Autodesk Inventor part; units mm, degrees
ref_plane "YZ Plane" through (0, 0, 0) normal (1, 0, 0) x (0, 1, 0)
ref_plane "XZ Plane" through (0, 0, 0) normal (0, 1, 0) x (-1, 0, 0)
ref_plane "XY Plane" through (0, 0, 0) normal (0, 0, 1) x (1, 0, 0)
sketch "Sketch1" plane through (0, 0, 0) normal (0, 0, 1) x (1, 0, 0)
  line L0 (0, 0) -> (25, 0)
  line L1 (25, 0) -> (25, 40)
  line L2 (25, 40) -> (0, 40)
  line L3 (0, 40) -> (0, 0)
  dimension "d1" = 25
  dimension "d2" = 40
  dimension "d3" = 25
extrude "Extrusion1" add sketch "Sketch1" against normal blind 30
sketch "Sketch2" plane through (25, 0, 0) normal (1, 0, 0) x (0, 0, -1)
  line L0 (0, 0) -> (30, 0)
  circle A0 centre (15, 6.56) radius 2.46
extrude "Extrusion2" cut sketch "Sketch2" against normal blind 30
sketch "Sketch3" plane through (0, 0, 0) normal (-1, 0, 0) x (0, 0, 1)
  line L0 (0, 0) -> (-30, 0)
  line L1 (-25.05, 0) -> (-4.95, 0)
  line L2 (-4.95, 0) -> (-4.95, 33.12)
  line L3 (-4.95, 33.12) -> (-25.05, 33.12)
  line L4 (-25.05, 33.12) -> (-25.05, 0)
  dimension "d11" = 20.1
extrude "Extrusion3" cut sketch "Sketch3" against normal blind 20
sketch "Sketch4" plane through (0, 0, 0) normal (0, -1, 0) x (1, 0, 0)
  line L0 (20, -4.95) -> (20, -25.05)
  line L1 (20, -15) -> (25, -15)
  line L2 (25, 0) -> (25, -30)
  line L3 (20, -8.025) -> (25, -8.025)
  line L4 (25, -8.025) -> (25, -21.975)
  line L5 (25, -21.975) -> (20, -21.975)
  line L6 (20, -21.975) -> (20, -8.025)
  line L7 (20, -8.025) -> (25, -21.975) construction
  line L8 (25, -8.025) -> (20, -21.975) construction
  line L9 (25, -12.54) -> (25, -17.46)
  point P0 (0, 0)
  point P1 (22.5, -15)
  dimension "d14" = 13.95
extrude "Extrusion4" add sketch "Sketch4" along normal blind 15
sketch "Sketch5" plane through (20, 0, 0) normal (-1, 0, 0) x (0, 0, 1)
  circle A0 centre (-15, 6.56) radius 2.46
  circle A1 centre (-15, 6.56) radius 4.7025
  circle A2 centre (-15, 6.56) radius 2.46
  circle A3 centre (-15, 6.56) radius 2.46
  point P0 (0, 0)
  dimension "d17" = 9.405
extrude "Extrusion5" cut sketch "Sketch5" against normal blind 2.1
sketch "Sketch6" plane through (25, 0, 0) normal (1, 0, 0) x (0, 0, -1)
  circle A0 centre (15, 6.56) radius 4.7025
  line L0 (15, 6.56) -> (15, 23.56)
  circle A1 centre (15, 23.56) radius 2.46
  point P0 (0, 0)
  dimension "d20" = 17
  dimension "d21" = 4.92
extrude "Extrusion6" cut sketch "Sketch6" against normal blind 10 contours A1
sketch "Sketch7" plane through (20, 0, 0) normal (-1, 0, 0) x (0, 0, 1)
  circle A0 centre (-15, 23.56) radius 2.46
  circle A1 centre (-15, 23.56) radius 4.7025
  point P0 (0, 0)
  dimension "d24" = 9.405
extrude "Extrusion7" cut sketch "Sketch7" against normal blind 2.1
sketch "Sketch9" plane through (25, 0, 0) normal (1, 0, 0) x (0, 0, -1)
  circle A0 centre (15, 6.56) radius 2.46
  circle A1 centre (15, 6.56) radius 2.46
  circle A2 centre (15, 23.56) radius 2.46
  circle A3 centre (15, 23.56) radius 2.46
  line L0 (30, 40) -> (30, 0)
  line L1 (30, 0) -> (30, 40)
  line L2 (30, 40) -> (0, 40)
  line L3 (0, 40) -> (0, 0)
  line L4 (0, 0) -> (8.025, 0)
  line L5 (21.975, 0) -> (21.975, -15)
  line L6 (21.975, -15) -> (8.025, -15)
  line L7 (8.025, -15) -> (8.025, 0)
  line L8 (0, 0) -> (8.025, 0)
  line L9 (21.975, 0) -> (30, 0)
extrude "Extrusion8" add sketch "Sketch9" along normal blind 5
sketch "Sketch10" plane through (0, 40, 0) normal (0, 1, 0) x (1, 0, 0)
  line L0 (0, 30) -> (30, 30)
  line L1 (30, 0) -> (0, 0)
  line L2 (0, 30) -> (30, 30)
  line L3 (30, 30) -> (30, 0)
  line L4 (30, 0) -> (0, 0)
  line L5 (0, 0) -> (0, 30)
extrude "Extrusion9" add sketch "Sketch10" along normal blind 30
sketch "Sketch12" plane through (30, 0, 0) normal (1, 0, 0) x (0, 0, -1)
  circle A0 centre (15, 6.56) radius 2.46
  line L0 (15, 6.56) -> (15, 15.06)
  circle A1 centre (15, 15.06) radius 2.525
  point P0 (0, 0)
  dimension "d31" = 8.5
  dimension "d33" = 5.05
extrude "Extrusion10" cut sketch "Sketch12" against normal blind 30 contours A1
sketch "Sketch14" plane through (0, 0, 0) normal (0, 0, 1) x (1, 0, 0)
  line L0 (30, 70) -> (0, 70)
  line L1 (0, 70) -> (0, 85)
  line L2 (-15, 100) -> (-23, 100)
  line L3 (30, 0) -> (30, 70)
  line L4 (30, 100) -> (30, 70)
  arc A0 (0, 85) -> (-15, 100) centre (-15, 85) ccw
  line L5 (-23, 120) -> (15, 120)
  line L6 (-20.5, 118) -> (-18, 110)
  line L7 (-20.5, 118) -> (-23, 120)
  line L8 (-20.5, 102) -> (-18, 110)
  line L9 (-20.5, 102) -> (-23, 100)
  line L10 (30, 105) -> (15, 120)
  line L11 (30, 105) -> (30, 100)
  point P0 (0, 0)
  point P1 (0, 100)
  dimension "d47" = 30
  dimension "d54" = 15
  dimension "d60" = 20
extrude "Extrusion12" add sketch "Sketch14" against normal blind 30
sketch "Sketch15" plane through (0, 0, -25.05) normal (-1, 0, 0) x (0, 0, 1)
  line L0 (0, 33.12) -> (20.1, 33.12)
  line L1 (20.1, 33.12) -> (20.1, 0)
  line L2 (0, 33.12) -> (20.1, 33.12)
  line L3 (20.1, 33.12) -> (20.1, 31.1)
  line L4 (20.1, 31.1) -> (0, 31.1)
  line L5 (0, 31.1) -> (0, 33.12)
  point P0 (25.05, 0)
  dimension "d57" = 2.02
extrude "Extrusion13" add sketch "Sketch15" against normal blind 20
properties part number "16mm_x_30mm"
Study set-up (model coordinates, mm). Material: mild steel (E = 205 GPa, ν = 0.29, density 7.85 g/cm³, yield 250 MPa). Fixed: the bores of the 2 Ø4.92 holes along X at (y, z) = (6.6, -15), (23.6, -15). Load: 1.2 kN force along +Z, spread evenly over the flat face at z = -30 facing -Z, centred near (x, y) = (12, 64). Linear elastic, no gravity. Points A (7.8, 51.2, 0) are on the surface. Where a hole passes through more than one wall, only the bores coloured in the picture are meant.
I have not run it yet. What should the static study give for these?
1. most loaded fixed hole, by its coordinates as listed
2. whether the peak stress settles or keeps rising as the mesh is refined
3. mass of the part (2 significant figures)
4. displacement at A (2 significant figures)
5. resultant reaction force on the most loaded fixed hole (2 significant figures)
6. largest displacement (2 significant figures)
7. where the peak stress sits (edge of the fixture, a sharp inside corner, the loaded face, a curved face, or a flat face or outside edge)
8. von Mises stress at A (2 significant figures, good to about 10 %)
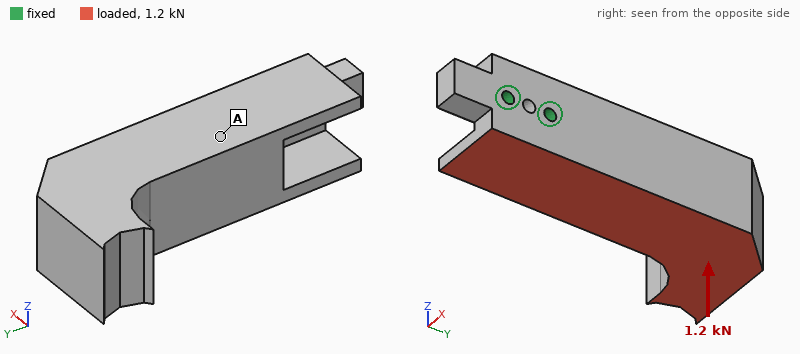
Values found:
(23.6, -15)
keeps rising
840 g
12 µm
3.2 kN
40 µm
edge of the fixture
6.0 MPa
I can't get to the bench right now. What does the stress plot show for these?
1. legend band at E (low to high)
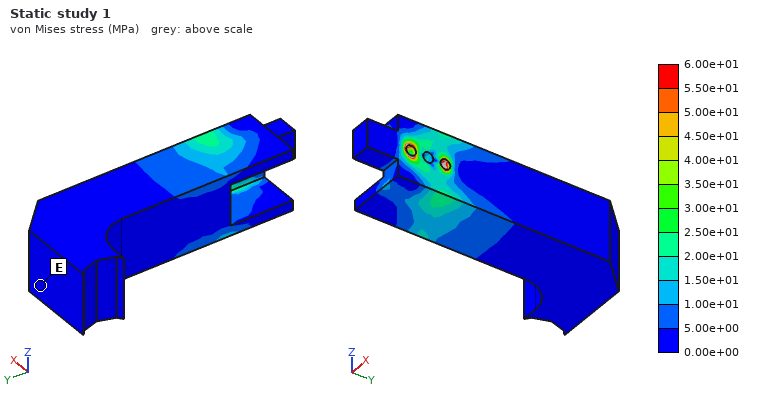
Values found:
0.00e+00 to 5.00e+00 MPa
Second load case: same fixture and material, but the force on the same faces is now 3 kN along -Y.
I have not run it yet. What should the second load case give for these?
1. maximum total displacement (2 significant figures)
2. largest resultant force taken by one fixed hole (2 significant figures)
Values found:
45 µm
3.1 kN
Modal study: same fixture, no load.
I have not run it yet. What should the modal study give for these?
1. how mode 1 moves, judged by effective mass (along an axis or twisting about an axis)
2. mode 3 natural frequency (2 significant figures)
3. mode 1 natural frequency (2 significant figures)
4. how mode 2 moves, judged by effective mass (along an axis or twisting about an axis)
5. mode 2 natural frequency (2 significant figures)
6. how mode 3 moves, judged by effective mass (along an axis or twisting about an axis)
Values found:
along X
3000 Hz
990 Hz
along Z
1200 Hz
twisting about Y
